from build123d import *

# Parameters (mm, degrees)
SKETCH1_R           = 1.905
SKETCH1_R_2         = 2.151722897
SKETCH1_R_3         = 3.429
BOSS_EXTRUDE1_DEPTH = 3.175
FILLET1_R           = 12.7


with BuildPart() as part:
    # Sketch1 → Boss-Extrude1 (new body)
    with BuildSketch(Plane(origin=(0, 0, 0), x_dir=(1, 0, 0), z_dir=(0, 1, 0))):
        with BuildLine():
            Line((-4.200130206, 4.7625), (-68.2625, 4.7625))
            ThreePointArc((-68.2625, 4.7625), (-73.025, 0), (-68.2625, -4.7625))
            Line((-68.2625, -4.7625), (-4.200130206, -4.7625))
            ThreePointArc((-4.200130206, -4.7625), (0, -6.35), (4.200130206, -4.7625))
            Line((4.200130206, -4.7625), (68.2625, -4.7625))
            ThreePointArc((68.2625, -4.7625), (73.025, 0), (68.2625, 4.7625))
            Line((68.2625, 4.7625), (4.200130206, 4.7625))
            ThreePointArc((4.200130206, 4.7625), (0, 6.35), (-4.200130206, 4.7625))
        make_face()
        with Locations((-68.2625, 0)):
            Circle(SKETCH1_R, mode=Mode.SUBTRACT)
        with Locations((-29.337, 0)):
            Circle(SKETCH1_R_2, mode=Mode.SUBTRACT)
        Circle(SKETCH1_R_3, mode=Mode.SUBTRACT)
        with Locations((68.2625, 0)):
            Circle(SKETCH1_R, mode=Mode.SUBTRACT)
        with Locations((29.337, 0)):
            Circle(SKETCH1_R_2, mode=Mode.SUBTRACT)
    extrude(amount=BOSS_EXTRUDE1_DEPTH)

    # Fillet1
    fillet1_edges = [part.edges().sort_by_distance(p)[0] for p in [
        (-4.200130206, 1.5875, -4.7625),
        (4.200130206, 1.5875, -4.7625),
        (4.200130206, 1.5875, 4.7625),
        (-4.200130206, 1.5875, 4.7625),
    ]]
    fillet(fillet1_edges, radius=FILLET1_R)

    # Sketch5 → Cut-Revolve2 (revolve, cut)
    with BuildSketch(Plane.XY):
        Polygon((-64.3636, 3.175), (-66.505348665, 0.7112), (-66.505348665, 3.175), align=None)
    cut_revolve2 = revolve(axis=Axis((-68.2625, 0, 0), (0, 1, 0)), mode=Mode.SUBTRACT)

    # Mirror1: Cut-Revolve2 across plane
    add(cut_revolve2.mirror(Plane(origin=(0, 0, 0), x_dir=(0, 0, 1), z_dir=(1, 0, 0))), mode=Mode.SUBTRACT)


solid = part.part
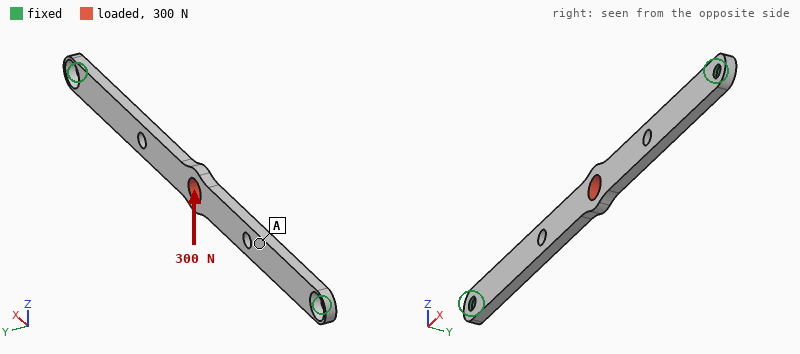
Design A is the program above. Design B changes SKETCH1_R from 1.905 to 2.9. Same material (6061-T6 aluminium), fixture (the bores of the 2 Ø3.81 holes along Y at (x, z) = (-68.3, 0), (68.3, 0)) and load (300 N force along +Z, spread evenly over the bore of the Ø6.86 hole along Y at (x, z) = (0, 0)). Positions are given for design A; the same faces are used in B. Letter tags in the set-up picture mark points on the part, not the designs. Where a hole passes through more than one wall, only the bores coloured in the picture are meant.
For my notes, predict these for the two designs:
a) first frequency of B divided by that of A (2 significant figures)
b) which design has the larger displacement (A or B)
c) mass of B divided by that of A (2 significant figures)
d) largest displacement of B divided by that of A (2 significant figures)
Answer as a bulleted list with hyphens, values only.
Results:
- 1.2
- A
- 0.99
- 0.76
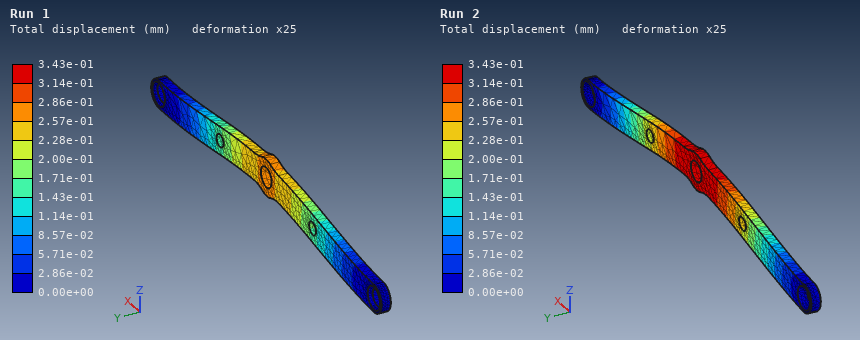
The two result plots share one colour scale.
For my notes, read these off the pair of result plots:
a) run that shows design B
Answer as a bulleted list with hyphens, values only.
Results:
- Run 1
